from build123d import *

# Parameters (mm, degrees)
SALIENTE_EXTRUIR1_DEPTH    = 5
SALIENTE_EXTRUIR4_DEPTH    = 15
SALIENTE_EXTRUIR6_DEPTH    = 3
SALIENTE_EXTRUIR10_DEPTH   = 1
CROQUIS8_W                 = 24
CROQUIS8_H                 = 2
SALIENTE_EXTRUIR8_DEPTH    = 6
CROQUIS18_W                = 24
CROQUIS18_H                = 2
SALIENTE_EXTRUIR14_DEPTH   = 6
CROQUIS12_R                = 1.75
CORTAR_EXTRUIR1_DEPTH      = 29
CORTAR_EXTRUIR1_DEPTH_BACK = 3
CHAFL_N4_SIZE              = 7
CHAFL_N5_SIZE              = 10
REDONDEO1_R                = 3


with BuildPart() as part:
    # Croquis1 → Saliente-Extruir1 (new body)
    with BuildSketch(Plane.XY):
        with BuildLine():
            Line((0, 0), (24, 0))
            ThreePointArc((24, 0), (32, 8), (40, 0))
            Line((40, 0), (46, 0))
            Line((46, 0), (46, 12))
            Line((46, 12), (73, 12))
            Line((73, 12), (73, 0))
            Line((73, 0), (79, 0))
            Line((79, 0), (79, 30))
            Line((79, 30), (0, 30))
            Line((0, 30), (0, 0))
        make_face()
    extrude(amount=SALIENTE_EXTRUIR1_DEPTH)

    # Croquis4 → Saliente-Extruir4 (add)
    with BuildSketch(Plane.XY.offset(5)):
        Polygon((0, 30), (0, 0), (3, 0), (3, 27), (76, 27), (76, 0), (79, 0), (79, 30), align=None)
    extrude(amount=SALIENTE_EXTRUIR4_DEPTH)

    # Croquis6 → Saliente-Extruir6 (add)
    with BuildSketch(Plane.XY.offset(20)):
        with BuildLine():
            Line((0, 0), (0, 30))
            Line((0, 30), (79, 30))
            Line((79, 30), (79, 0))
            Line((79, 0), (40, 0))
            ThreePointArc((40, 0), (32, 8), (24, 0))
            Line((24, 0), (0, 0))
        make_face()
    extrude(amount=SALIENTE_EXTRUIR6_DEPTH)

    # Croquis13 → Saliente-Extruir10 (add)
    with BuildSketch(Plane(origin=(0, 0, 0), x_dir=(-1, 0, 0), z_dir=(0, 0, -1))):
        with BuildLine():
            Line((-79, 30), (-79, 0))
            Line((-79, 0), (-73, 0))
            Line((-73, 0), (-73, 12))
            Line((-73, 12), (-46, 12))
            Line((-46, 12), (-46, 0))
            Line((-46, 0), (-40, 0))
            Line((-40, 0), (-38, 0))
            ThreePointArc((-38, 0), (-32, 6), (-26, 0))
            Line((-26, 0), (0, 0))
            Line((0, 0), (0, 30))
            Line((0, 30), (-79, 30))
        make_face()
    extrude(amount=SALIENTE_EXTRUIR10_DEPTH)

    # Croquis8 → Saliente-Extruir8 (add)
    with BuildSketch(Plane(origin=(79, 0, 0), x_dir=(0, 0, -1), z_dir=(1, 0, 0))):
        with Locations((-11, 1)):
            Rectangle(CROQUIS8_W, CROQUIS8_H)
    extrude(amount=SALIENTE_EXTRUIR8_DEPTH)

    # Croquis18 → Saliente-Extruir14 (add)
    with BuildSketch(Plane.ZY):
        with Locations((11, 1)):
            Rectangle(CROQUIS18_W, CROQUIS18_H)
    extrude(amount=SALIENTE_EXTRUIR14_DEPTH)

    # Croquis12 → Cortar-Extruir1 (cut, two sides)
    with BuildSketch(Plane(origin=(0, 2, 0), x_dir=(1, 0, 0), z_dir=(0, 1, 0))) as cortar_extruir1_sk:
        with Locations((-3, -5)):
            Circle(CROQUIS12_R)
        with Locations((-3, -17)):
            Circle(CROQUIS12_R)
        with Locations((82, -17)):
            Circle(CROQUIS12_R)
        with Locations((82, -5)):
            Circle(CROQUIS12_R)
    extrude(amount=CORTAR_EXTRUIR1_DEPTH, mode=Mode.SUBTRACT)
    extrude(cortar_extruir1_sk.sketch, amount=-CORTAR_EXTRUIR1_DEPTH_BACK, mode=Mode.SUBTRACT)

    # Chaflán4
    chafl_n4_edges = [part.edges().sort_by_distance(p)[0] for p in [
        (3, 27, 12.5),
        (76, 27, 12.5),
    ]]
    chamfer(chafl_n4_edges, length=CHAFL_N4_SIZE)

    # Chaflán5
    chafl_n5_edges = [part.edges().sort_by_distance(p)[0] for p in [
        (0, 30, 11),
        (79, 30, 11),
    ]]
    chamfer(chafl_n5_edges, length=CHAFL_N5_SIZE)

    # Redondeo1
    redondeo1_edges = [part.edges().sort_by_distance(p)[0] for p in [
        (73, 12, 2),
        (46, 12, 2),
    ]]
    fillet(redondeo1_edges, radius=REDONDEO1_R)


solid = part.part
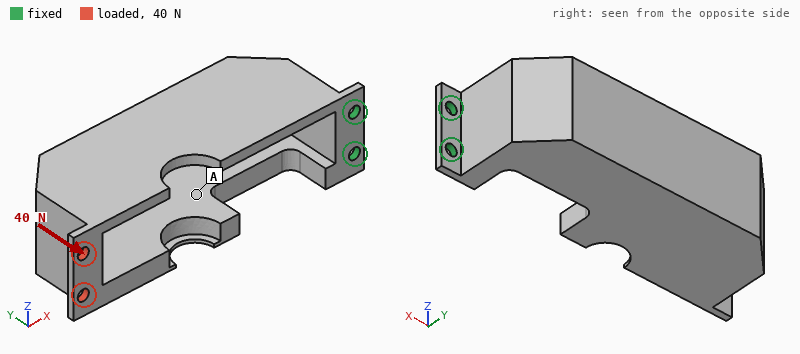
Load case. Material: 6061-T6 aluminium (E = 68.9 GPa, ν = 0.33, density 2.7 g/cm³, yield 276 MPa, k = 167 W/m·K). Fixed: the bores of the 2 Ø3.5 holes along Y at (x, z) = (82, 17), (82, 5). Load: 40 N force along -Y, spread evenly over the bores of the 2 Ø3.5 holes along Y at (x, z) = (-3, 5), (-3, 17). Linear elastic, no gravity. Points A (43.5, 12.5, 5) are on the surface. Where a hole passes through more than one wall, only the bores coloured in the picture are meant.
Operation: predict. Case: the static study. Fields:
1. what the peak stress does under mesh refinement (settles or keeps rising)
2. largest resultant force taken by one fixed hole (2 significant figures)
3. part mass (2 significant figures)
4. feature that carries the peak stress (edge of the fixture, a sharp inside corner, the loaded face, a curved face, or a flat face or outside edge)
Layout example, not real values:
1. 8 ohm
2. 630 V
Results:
1. keeps rising
2. 80 N
3. 63 g
4. edge of the fixture
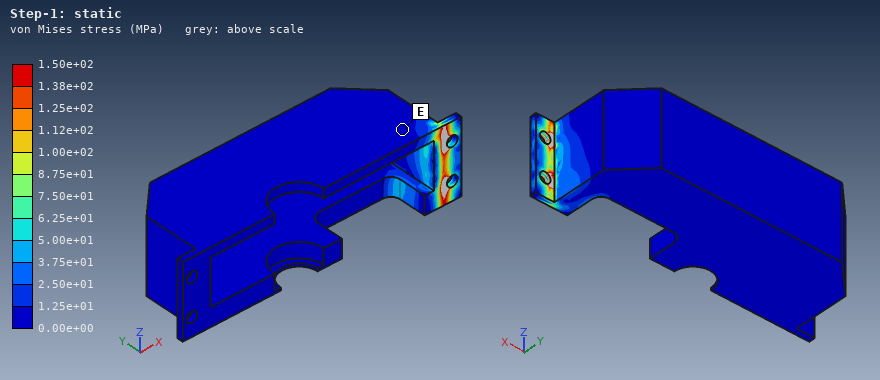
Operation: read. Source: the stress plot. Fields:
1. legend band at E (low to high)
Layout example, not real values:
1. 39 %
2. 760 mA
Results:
1. 0.00e+00 to 1.25e+01 MPa
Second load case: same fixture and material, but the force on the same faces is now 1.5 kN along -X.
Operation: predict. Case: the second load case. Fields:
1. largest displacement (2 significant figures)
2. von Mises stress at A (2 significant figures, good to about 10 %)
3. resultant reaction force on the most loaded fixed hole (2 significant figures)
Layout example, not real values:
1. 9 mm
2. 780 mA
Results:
1. 0.59 mm
2. 31 MPa
3. 820 N
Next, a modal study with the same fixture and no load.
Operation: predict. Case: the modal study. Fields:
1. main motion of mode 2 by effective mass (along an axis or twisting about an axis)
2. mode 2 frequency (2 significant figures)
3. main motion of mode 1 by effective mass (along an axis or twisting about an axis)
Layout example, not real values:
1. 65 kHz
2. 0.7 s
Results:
1. along Z
2. 560 Hz
3. along Y
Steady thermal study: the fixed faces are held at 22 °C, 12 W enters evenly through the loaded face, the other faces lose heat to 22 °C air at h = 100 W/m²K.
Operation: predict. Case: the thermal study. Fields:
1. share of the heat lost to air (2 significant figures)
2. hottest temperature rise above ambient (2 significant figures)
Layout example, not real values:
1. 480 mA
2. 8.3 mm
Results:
1. 81 %
2. 28 K
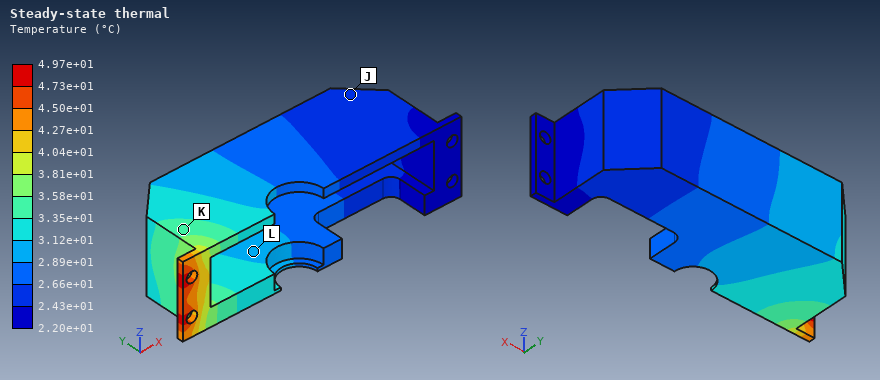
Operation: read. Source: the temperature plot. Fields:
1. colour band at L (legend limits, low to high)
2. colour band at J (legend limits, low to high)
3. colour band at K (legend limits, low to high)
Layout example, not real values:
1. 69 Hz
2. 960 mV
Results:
1. 2.89e+01 to 3.12e+01 °C
2. 2.43e+01 to 2.66e+01 °C
3. 3.35e+01 to 3.58e+01 °C
